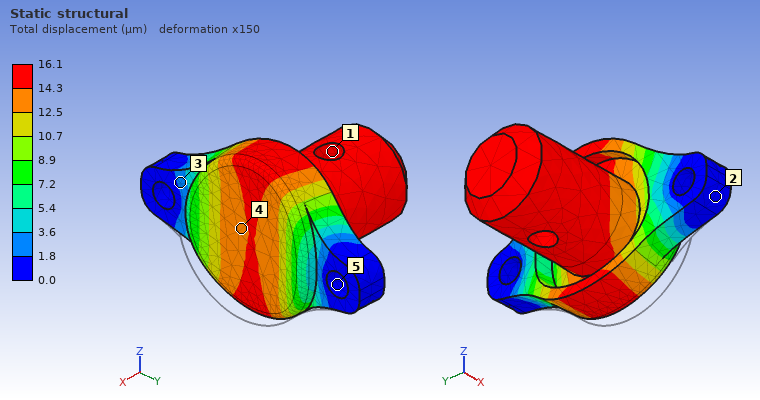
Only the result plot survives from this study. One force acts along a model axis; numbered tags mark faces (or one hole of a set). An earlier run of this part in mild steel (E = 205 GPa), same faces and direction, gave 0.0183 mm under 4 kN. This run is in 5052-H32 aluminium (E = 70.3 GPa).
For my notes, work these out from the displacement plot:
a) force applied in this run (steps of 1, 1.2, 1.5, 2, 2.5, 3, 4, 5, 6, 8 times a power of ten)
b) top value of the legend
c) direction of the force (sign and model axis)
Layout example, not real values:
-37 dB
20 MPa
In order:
1.2 kN
16.1 µm
-X
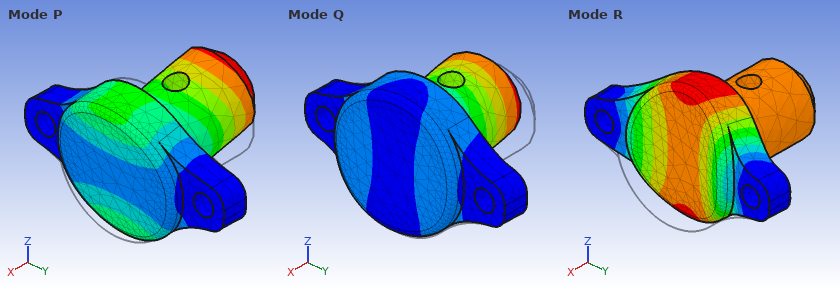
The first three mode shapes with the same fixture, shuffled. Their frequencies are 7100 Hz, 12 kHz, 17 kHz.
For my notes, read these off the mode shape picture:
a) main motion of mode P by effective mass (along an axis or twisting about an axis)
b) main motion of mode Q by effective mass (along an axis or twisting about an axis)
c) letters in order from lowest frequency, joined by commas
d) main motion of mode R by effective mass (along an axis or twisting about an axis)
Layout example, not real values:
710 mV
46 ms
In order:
along Z
along Y
P, Q, R
along X
